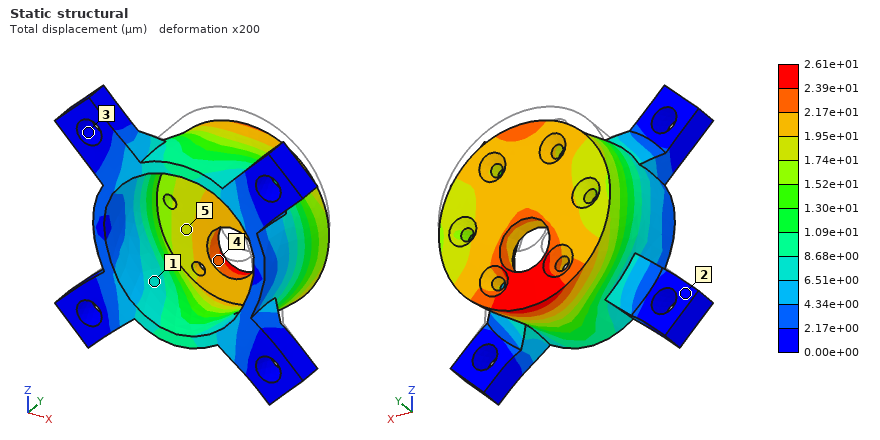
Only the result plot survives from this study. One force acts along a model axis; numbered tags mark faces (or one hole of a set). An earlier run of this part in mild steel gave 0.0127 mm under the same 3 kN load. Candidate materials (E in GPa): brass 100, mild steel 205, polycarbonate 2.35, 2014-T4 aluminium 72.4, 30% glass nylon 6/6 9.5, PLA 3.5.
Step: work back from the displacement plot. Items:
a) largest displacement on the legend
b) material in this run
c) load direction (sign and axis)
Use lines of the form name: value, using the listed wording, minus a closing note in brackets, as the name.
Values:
largest displacement on the legend: 2.61e+01 µm
material in this run: brass
load direction: -Z
